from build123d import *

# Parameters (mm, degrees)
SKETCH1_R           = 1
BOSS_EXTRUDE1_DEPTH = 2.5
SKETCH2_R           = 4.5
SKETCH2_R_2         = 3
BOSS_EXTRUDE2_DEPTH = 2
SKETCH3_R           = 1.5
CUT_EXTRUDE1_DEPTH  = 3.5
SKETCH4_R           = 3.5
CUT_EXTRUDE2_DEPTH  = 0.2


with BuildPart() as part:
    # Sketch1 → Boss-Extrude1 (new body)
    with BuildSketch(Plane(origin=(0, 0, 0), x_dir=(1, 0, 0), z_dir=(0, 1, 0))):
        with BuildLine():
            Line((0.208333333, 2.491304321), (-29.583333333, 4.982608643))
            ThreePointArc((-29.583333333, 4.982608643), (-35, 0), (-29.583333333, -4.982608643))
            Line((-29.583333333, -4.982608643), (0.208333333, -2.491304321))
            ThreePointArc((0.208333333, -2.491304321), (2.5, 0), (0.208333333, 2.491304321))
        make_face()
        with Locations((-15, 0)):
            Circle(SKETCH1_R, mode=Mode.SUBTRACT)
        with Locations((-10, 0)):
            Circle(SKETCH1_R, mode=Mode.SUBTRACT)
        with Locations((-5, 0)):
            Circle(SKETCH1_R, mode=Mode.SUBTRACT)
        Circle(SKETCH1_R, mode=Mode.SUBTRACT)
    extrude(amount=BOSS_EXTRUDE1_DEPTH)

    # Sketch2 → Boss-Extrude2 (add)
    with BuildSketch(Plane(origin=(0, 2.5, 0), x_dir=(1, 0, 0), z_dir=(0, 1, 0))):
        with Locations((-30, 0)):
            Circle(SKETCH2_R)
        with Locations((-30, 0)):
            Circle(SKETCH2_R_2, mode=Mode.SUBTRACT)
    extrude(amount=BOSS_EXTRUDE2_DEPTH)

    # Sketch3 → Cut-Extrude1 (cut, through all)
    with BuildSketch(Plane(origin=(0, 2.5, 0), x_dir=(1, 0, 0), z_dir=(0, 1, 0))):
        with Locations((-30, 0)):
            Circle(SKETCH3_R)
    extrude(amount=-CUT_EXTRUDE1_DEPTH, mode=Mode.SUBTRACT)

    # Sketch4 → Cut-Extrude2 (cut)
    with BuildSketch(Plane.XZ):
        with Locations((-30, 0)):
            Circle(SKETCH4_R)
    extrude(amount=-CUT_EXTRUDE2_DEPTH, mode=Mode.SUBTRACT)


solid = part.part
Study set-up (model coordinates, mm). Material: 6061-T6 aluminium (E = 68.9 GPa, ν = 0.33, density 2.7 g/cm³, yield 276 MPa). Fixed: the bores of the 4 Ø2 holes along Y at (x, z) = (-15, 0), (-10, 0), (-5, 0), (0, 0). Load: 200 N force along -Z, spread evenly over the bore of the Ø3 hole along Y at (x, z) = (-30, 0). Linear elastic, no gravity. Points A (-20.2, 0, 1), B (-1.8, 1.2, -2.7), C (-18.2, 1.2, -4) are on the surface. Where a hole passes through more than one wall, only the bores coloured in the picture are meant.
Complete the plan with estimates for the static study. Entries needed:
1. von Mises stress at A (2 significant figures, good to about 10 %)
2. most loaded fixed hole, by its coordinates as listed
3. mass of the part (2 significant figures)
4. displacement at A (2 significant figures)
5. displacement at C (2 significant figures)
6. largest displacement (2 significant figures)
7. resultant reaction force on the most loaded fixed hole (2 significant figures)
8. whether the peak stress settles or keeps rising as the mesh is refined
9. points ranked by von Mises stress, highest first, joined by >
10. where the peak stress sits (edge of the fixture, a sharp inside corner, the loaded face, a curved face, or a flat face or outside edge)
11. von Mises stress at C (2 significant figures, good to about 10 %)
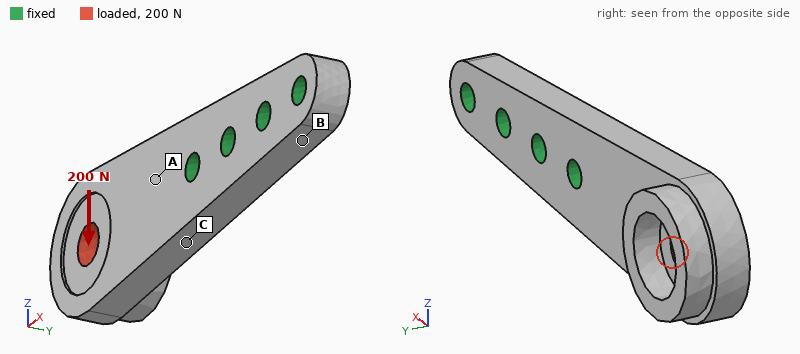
31 MPa
(-15, 0)
1.9 g
14 µm
13 µm
77 µm
490 N
keeps rising
C > A > B
edge of the fixture
87 MPa
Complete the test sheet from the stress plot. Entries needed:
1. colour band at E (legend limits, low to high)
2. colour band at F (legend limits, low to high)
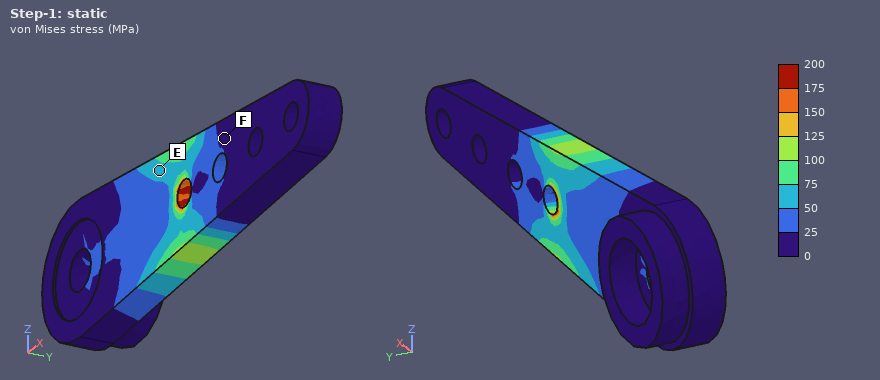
50 to 75 MPa
0 to 25 MPa
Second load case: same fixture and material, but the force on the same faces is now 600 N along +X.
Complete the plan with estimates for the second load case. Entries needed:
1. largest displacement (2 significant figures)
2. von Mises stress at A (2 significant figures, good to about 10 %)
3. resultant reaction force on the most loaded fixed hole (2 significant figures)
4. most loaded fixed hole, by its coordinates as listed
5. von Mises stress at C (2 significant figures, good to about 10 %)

14 µm
25 MPa
490 N
(-15, 0)
22 MPa
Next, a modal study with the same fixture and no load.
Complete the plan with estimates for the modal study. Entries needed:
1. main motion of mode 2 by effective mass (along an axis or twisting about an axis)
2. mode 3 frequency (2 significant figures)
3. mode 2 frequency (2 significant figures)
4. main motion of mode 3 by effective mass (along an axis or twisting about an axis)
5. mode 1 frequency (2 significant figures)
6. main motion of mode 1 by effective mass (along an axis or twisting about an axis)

along Z
17 kHz
10 kHz
twisting about X
4700 Hz
along Y
